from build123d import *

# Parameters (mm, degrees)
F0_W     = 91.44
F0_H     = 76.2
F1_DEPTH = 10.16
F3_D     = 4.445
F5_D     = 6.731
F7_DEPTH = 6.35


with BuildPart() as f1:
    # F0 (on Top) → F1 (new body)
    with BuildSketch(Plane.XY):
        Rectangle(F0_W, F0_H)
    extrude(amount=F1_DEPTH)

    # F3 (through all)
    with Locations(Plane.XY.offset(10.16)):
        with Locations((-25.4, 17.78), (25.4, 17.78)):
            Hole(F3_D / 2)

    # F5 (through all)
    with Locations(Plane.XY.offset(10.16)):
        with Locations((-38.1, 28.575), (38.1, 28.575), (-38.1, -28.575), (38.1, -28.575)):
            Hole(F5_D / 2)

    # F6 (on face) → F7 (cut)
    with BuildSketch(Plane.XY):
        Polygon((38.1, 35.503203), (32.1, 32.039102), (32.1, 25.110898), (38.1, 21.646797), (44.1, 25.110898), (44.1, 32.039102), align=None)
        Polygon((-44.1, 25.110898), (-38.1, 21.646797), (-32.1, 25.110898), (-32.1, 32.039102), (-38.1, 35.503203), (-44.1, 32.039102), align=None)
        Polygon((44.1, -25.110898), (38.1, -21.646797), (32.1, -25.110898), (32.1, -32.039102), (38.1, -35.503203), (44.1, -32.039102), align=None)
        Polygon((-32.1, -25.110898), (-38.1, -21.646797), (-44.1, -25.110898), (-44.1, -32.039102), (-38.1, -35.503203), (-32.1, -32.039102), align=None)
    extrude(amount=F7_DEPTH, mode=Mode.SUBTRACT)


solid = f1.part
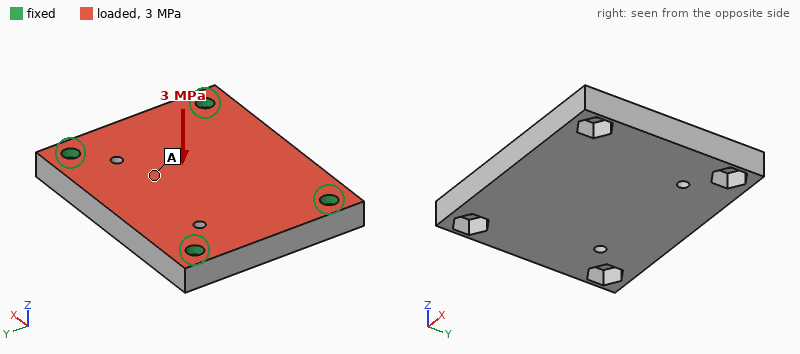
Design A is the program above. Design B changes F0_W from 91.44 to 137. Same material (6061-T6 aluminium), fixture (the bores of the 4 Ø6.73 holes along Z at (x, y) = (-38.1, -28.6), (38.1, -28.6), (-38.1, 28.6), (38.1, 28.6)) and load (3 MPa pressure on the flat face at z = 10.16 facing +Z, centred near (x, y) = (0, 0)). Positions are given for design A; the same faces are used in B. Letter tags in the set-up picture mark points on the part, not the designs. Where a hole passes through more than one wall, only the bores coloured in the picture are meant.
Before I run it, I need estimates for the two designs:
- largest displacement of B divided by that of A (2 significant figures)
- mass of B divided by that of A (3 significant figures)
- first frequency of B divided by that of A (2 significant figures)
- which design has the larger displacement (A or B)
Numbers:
1.1
1.53
0.80
B
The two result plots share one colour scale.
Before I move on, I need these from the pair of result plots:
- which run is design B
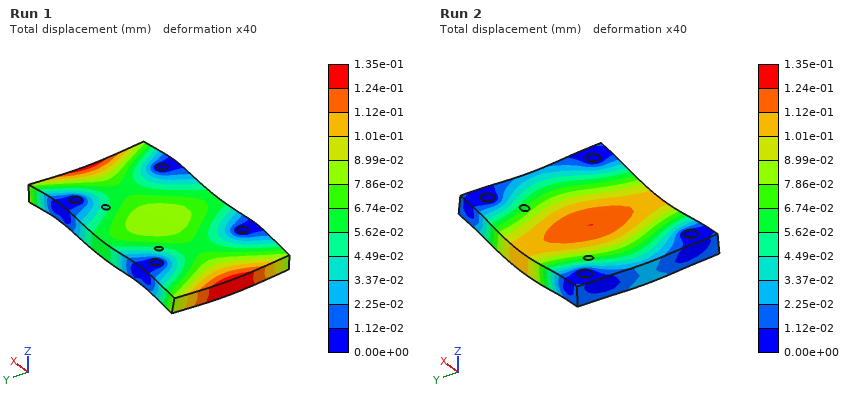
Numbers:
Run 1
